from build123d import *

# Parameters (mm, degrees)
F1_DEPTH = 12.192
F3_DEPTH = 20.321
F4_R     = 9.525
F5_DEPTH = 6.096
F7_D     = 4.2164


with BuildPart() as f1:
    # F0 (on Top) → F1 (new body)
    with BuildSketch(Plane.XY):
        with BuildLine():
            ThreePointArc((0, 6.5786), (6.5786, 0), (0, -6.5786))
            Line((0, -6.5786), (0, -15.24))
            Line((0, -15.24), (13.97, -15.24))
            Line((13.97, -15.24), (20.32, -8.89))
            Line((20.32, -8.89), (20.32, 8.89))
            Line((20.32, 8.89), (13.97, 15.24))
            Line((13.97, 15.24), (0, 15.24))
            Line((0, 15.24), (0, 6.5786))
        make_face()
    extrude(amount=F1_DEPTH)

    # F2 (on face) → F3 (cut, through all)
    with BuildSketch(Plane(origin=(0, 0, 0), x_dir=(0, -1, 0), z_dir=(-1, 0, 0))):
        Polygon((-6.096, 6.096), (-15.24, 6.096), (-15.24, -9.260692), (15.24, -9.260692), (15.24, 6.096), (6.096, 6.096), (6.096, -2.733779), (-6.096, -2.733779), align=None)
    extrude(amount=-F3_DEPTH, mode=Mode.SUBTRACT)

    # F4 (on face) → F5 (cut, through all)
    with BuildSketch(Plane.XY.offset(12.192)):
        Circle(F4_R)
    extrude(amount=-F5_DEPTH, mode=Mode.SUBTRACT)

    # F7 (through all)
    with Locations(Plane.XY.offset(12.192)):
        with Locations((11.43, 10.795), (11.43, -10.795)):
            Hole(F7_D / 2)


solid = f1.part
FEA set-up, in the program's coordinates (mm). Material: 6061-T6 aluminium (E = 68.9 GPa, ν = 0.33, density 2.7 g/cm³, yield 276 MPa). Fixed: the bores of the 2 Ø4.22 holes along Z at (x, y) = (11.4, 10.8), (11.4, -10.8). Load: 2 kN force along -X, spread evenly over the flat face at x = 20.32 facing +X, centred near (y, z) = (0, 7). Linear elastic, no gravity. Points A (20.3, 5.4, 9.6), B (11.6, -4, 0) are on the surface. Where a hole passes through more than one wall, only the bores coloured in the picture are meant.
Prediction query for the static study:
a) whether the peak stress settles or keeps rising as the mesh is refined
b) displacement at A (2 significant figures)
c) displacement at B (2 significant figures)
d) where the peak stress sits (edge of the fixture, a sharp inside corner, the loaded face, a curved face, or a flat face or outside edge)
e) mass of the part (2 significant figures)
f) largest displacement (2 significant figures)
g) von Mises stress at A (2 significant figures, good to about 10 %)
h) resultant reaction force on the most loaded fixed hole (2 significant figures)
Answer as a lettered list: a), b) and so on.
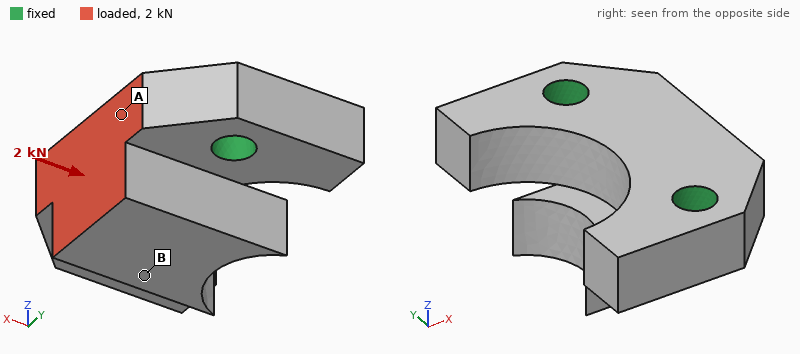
a) keeps rising
b) 6.6 µm
c) 12 µm
d) edge of the fixture
e) 9.7 g
f) 15 µm
g) 24 MPa
h) 1.1 kN
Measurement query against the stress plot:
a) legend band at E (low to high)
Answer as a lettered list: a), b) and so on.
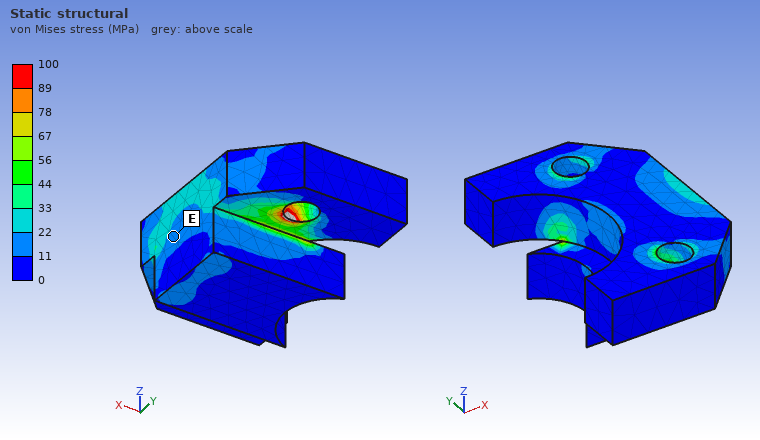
a) 11 to 22 MPa
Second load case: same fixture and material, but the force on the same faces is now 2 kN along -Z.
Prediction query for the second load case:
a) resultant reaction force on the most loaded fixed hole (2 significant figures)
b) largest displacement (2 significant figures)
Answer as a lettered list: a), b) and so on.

a) 1.0 kN
b) 36 µm
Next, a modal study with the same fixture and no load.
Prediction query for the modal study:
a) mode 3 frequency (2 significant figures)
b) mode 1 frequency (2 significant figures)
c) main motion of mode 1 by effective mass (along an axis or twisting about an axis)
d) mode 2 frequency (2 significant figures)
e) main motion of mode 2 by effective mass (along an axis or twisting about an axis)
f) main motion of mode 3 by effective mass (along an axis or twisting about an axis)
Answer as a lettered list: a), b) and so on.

a) 44 kHz
b) 24 kHz
c) along X
d) 41 kHz
e) along Z
f) along Z
